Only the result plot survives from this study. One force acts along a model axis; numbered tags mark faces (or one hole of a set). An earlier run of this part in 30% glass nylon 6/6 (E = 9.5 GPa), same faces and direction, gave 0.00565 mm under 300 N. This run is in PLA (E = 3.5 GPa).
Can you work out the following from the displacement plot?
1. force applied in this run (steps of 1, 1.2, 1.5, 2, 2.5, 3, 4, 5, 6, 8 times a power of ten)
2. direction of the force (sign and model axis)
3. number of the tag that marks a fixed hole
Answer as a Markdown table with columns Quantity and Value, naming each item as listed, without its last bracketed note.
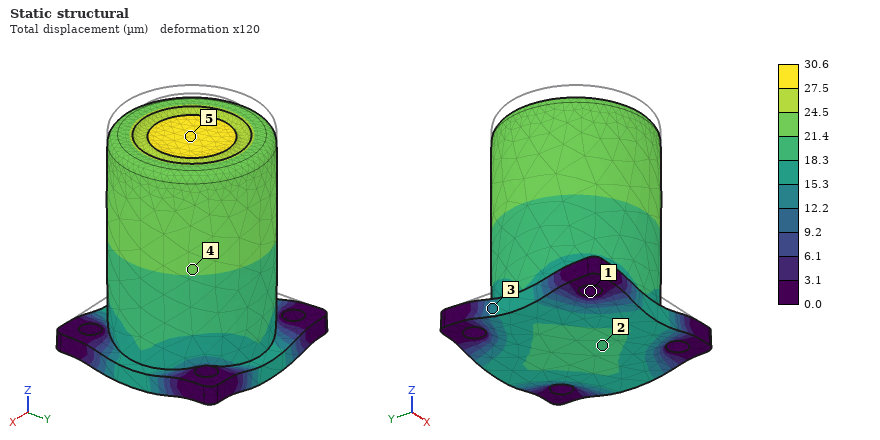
| Quantity | Value |
|---|---|
| force applied in this run | 600 N |
| direction of the force | -Z |
| number of the tag that marks a fixed hole | 1 |
